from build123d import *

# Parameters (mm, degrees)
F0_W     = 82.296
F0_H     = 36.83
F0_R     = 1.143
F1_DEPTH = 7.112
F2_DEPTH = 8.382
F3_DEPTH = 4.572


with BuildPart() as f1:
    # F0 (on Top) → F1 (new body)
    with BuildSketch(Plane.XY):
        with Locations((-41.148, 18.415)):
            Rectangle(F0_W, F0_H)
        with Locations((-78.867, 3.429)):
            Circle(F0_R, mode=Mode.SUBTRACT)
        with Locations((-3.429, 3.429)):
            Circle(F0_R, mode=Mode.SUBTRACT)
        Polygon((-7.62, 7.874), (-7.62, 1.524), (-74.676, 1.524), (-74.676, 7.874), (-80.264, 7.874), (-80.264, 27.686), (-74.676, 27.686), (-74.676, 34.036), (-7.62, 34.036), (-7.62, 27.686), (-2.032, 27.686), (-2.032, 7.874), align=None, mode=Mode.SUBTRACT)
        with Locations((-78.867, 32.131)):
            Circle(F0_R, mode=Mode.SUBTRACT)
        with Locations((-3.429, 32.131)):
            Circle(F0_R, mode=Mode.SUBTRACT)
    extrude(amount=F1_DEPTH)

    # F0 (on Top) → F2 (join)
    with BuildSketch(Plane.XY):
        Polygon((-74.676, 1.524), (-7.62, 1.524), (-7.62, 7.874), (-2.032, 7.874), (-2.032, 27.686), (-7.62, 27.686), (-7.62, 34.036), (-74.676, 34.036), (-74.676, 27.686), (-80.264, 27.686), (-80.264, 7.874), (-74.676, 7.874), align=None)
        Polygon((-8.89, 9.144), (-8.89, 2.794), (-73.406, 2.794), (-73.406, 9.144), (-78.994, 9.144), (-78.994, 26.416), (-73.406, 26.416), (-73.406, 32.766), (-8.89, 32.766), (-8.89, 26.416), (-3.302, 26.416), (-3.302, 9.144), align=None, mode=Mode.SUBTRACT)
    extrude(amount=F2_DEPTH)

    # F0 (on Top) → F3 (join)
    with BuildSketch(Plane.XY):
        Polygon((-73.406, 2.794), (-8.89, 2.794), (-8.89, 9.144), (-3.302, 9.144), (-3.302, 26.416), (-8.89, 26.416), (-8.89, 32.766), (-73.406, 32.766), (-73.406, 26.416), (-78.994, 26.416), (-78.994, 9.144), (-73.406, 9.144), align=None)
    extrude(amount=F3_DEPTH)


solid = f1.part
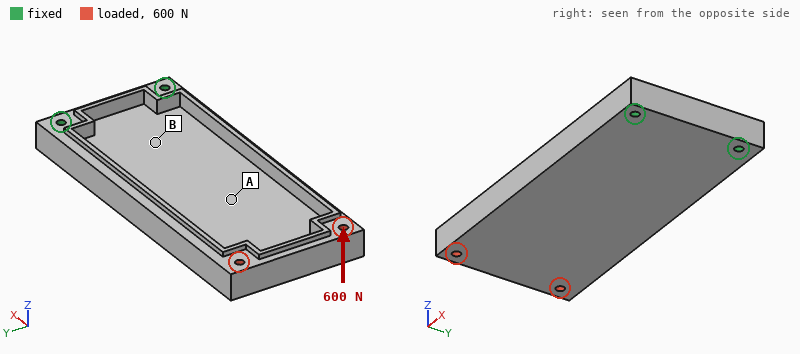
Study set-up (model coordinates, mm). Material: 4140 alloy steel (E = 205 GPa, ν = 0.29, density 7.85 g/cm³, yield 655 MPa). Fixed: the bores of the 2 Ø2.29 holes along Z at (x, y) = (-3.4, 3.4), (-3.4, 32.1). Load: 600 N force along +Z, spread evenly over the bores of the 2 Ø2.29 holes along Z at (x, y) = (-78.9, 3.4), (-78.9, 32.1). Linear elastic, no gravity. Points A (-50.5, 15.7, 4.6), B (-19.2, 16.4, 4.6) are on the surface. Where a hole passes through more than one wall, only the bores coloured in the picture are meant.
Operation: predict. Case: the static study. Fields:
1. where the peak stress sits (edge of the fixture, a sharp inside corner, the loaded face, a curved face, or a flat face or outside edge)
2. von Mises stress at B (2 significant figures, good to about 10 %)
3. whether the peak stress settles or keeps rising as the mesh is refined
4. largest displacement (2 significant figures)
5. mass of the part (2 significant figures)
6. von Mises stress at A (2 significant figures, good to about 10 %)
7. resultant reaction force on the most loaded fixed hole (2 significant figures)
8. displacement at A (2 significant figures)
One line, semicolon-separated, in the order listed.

edge of the fixture; 120 MPa; keeps rising; 0.83 mm; 130 g; 54 MPa; 680 N; 0.37 mm
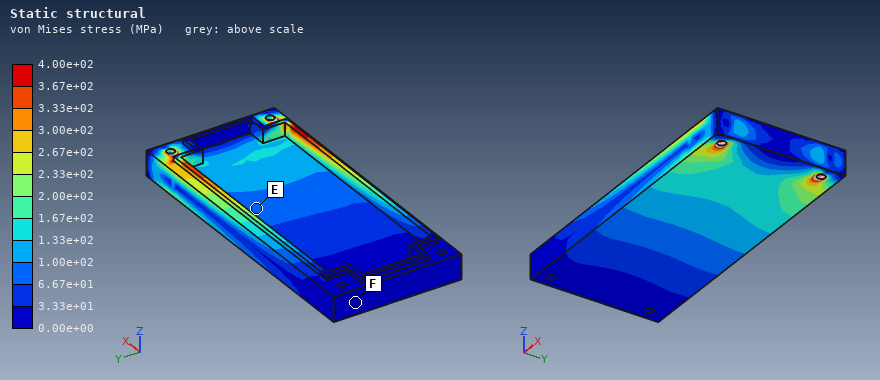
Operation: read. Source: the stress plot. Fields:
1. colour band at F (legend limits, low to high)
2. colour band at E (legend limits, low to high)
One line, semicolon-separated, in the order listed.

0.00e+00 to 3.33e+01 MPa; 6.67e+01 to 1.00e+02 MPa
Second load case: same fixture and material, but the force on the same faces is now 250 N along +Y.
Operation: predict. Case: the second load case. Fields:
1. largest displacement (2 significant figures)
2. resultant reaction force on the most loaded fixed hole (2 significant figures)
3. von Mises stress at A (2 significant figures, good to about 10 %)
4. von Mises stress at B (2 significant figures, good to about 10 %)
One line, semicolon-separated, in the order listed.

14 µm; 660 N; 6.7 MPa; 5.9 MPa
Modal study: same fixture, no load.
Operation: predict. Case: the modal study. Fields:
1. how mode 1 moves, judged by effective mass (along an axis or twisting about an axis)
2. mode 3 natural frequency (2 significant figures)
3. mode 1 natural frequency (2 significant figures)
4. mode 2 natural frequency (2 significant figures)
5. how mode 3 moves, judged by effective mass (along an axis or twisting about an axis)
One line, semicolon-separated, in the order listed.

along Z; 4200 Hz; 740 Hz; 2600 Hz; along Y
